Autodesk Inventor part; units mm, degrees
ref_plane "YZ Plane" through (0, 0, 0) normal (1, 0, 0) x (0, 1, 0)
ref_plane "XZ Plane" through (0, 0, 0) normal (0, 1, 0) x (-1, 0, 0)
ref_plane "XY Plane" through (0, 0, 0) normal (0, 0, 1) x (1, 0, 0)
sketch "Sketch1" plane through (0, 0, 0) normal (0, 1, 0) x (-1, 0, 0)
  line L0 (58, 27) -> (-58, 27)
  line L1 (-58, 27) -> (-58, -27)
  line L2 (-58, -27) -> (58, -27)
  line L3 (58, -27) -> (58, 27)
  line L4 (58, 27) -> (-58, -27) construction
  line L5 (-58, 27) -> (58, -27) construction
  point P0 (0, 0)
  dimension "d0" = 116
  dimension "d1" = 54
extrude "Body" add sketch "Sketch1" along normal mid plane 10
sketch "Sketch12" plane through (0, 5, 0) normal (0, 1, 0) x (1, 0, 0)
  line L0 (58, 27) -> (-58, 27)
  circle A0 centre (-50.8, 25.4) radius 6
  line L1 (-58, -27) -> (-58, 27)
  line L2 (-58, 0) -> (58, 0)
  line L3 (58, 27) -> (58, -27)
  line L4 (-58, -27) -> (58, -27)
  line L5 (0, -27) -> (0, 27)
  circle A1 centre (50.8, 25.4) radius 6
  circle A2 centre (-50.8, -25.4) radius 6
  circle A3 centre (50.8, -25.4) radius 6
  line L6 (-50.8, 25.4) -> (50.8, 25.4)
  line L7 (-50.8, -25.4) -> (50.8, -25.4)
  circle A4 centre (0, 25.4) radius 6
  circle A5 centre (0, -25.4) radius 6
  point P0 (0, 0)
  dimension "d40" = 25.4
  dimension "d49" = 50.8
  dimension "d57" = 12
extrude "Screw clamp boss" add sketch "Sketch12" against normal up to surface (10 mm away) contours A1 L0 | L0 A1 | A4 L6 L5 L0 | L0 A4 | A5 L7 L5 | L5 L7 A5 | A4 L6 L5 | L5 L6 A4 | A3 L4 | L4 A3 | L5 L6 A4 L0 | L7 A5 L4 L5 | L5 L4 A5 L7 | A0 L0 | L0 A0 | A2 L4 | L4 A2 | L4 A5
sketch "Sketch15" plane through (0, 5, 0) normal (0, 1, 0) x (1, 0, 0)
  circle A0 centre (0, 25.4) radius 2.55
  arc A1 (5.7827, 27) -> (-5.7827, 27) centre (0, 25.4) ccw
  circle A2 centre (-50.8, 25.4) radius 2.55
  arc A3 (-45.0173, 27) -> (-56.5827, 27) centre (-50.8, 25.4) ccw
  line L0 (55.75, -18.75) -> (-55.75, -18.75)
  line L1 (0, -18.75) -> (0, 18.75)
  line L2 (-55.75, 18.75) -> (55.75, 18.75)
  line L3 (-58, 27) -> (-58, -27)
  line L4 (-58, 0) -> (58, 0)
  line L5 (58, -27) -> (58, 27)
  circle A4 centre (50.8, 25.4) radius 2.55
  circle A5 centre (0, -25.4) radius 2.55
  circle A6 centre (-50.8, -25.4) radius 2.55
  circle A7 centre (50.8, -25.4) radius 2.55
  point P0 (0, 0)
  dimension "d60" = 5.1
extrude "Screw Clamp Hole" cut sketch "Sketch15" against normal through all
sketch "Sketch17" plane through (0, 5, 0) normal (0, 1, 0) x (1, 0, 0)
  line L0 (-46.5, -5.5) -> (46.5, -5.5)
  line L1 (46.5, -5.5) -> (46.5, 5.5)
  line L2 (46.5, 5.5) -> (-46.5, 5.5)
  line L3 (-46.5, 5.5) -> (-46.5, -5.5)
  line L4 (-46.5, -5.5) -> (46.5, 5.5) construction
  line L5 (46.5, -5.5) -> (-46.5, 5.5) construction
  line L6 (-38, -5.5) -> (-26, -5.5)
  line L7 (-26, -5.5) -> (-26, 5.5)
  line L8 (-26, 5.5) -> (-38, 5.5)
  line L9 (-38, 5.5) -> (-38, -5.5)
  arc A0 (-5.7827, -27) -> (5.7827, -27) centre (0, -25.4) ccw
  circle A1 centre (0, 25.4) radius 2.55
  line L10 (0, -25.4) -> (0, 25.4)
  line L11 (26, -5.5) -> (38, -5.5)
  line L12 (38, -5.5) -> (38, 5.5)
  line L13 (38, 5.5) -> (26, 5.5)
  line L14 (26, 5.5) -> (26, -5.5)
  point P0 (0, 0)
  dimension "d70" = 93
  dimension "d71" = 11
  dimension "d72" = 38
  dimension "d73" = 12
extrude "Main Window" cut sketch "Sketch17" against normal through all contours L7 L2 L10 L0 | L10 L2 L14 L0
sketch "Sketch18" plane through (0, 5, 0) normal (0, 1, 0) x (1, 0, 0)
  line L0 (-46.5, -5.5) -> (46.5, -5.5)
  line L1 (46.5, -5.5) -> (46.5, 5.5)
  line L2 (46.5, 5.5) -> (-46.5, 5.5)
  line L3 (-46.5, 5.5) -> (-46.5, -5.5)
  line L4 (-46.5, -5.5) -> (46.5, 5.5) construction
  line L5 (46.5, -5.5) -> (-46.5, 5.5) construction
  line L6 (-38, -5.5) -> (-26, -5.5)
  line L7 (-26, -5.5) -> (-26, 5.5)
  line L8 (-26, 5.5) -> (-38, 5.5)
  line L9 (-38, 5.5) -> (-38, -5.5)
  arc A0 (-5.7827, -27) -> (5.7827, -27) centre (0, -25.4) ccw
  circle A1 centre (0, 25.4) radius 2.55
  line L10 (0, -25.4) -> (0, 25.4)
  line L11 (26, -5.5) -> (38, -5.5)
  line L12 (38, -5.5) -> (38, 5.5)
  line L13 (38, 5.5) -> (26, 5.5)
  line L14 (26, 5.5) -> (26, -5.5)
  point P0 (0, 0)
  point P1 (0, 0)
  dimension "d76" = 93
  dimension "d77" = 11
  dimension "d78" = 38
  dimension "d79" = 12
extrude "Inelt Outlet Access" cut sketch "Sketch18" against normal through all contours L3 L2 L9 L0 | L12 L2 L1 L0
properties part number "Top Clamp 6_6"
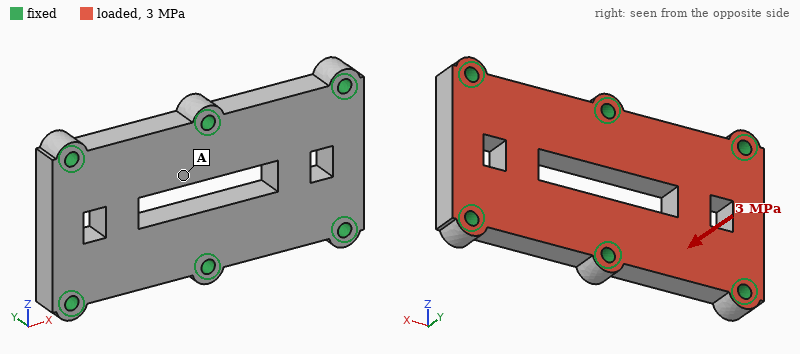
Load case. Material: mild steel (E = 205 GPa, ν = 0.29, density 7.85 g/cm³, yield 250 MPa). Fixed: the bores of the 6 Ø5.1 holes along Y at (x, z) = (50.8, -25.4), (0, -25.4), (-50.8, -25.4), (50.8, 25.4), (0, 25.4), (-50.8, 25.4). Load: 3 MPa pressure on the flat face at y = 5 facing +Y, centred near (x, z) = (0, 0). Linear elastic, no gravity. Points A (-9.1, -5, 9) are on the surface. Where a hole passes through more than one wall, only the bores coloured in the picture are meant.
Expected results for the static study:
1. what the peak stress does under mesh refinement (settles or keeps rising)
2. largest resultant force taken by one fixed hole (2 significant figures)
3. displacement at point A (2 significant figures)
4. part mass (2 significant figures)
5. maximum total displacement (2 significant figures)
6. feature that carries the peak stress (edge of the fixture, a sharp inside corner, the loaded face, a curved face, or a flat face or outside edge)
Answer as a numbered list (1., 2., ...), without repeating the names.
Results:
1. keeps rising
2. 3.6 kN
3. 8.9 µm
4. 440 g
5. 12 µm
6. edge of the fixture
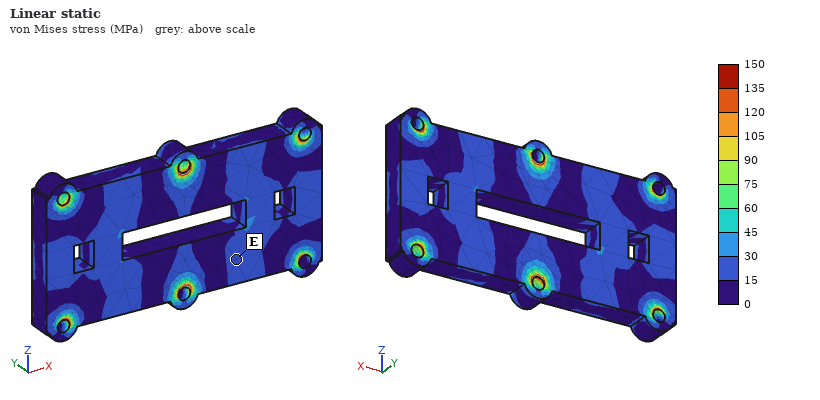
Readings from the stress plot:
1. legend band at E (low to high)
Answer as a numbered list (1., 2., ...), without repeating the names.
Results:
1. 15 to 30 MPa
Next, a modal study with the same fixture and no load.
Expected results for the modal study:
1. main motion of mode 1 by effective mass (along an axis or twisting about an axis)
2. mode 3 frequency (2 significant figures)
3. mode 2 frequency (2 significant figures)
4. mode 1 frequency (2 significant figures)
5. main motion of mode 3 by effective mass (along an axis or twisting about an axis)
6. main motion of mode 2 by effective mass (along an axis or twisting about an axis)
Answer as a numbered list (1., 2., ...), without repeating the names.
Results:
1. along Y
2. 17 kHz
3. 12 kHz
4. 11 kHz
5. twisting about X
6. twisting about Z
